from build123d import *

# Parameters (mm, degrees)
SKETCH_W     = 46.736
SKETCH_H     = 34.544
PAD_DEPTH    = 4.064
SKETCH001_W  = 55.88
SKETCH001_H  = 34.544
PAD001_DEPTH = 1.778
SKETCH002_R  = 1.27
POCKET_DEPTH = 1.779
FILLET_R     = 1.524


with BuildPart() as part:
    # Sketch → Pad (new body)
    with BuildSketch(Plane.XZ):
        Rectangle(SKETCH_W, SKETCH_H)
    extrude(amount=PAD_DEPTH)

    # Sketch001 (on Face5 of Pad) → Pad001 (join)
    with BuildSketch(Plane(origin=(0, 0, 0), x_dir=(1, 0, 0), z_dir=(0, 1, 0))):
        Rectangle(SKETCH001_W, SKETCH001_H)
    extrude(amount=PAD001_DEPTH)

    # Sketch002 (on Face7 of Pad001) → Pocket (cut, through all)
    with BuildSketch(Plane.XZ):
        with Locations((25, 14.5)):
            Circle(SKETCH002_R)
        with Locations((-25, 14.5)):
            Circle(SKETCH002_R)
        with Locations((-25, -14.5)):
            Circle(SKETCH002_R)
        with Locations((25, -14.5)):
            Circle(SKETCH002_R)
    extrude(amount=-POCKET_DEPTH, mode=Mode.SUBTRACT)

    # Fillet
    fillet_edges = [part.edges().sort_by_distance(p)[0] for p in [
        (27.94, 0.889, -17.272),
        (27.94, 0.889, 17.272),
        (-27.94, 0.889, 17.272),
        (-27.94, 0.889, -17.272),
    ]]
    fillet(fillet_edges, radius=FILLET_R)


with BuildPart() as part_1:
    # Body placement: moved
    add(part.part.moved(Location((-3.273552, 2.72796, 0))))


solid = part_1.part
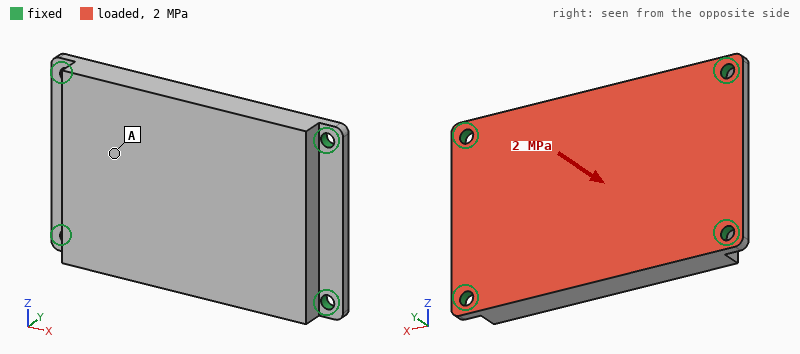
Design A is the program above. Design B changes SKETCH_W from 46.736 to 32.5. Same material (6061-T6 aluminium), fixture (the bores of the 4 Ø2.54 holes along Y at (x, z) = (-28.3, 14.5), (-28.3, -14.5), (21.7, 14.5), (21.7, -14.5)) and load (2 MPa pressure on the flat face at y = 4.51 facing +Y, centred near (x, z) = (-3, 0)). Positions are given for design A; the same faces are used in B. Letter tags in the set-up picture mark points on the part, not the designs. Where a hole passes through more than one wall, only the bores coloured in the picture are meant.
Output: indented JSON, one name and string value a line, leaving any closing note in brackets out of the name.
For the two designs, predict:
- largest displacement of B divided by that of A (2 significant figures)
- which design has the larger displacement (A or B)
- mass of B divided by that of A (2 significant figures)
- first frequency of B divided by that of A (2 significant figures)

{
  "largest displacement of B divided by that of A": "2.5",
  "which design has the larger displacement": "B",
  "mass of B divided by that of A": "0.80",
  "first frequency of B divided by that of A": "0.64"
}
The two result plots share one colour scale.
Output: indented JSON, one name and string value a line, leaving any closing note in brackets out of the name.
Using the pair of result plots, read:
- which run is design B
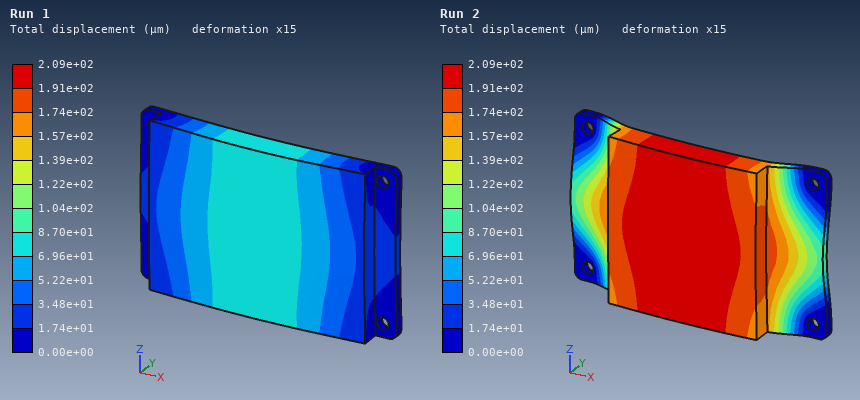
{
  "which run is design B": "Run 2"
}
